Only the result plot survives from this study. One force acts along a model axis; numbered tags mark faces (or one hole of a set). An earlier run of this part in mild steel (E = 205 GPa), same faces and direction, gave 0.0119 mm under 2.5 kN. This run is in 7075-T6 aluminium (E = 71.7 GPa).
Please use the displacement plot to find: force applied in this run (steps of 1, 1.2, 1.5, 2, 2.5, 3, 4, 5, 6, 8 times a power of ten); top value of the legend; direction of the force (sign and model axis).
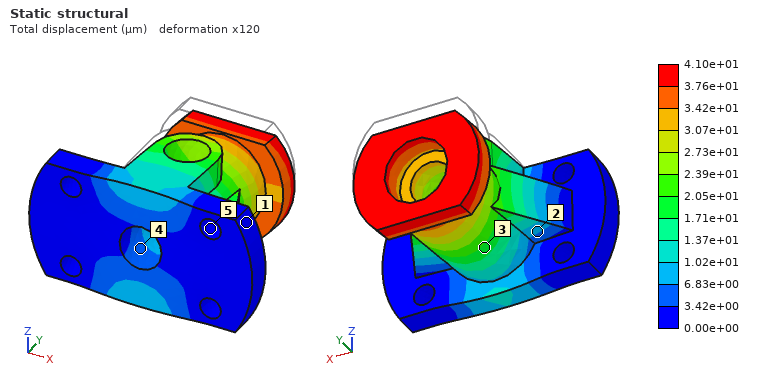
3 kN
4.10e+01 µm
-Z
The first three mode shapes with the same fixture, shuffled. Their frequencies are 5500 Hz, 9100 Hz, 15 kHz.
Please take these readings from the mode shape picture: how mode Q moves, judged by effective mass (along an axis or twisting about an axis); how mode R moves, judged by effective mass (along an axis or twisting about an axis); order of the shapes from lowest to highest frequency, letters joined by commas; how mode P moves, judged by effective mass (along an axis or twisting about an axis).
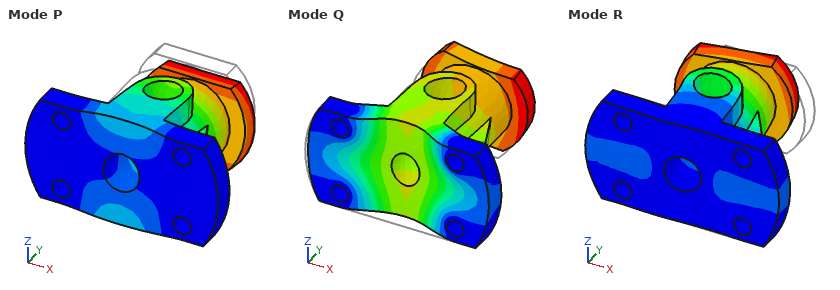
along Y
along X
P, R, Q
along Z
